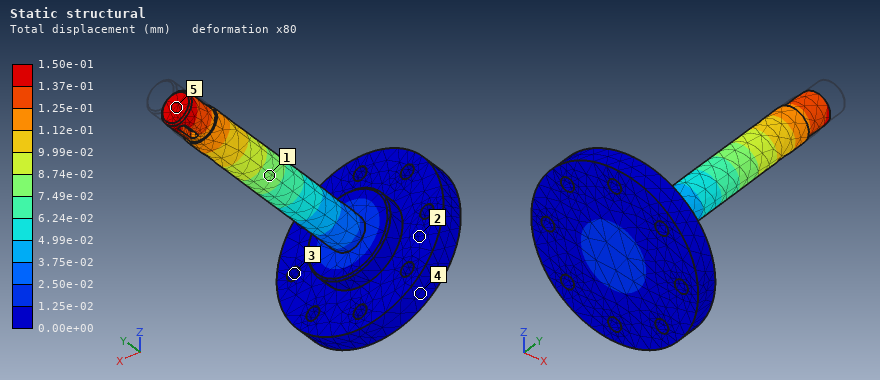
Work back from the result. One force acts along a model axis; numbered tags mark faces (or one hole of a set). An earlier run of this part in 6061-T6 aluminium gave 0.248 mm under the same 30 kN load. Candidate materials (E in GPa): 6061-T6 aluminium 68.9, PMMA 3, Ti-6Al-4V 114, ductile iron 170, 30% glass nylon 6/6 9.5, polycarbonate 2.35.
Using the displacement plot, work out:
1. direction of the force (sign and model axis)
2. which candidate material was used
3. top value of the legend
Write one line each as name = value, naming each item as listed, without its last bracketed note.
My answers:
direction of the force = -Y
which candidate material was used = Ti-6Al-4V
top value of the legend = 1.50e-01 mm
